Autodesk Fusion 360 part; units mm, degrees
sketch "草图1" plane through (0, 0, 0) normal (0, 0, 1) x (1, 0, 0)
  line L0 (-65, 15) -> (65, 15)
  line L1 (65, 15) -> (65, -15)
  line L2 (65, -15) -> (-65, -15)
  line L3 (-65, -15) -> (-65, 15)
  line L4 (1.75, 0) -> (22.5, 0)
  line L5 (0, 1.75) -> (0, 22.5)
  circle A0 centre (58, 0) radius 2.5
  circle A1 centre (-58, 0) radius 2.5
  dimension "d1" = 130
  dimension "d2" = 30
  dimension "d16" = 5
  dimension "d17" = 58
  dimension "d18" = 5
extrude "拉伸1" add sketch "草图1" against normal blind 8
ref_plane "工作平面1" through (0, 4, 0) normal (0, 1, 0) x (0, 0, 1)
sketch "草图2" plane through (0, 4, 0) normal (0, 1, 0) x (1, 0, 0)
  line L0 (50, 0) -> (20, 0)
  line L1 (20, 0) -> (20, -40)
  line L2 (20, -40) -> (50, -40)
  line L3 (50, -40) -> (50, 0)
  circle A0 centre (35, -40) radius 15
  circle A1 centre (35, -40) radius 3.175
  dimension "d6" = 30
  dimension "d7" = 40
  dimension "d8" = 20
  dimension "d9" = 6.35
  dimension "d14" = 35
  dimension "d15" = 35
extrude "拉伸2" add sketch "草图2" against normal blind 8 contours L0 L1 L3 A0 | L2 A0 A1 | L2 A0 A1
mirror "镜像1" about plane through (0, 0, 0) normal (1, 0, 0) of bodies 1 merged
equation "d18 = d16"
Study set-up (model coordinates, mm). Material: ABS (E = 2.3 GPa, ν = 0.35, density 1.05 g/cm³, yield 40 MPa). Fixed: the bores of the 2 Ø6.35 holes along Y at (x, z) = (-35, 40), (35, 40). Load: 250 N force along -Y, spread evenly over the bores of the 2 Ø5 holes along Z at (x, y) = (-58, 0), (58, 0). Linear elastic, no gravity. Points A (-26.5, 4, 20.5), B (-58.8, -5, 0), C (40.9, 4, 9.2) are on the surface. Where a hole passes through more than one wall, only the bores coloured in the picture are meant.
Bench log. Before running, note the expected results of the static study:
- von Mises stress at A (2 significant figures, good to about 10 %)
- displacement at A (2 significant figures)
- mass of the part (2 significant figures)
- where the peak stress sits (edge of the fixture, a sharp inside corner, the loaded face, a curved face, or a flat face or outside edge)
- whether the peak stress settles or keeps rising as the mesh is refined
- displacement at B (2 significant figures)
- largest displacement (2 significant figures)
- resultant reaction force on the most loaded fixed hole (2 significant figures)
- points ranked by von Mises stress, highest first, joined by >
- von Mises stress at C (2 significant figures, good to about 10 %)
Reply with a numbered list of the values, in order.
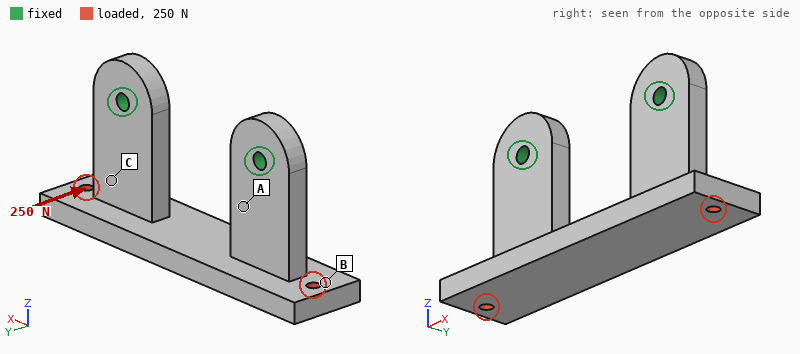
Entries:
1. 9.2 MPa
2. 0.33 mm
3. 58 g
4. edge of the fixture
5. keeps rising
6. 1.2 mm
7. 1.6 mm
8. 130 N
9. A > C > B
10. 5.0 MPa
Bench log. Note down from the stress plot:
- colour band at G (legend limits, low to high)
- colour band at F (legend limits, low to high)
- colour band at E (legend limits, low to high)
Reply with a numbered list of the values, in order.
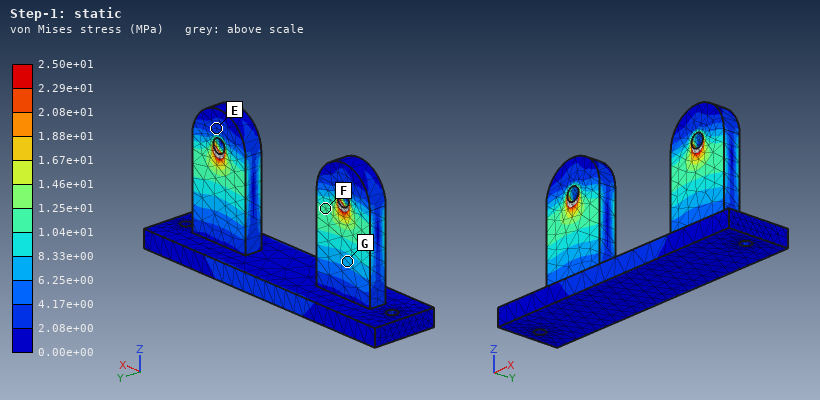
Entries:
1. 6.25e+00 to 8.33e+00 MPa
2. 1.04e+01 to 1.25e+01 MPa
3. 2.08e+00 to 4.17e+00 MPa
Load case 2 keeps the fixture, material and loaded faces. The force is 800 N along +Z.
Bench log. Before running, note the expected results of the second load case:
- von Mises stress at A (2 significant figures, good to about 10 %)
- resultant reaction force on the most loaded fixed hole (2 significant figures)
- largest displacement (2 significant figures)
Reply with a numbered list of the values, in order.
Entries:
1. 1.2 MPa
2. 450 N
3. 0.44 mm
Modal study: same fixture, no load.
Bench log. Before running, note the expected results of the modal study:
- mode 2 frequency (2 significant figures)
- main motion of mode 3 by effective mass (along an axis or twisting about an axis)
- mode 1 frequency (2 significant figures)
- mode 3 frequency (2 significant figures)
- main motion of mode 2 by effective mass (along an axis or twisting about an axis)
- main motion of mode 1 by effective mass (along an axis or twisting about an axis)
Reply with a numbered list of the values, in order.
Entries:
1. 560 Hz
2. along X
3. 360 Hz
4. 870 Hz
5. twisting about Z
6. along Y
